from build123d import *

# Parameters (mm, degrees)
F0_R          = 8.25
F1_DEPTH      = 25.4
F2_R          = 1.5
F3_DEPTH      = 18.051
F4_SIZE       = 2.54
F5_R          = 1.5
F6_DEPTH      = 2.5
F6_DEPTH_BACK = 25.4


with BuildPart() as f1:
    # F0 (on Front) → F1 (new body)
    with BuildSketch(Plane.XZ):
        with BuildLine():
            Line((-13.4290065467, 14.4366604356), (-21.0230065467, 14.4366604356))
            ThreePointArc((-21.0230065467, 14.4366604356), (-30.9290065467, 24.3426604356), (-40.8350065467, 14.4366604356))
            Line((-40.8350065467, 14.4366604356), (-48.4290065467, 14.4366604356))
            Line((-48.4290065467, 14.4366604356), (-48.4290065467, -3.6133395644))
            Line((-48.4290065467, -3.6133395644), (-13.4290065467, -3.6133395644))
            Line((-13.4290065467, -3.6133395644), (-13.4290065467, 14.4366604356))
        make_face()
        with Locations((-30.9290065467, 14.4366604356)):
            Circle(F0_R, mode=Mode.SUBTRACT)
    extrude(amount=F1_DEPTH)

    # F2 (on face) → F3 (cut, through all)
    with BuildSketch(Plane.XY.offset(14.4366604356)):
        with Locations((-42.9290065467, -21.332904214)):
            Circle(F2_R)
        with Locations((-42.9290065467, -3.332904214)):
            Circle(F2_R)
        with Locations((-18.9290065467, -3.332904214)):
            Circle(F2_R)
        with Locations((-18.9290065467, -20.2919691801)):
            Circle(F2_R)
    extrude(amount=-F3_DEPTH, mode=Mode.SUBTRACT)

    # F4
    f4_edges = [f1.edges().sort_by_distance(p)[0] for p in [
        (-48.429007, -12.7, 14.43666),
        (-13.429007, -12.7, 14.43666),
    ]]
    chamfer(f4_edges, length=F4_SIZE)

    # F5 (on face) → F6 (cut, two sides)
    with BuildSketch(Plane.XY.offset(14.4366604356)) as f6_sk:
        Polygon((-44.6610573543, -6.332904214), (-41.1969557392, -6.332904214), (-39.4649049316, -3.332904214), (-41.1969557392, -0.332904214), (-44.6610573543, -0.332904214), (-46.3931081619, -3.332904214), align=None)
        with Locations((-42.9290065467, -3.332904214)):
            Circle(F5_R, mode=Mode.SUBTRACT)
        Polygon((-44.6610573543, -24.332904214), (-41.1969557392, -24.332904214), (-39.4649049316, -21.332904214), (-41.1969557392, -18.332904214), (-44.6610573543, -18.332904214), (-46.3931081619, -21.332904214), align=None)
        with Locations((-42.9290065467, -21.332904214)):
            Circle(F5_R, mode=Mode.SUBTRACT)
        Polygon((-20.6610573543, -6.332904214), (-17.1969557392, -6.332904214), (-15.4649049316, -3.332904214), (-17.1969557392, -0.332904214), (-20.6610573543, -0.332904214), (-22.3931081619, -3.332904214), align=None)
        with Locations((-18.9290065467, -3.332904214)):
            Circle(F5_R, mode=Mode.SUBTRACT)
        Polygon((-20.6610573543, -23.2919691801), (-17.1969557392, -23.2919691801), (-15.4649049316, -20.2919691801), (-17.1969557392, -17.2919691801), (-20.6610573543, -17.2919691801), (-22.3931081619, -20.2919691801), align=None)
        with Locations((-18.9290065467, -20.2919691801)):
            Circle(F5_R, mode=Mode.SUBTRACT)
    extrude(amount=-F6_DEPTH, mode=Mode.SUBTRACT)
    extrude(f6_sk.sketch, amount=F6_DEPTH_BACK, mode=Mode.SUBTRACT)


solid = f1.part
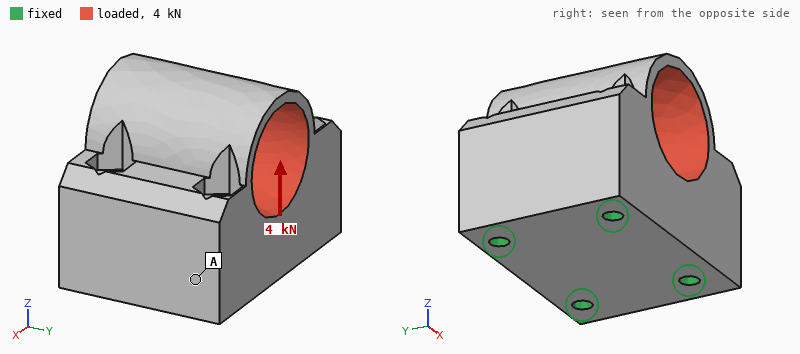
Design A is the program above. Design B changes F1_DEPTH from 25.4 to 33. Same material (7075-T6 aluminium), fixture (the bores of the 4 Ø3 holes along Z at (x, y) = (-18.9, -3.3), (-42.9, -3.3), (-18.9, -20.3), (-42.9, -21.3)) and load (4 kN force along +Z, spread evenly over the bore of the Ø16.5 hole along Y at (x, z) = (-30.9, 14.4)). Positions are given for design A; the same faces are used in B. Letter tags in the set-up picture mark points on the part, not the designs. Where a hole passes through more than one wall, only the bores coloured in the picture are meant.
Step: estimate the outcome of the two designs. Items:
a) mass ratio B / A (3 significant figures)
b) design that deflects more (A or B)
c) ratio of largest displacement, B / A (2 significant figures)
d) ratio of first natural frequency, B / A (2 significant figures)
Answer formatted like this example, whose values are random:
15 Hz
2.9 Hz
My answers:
1.32
A
0.73
1.0
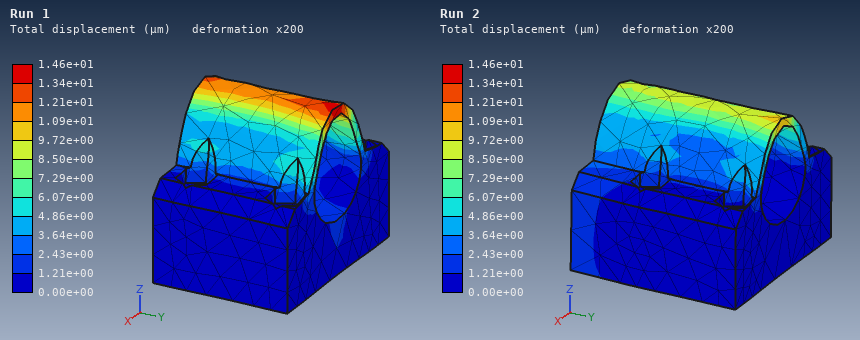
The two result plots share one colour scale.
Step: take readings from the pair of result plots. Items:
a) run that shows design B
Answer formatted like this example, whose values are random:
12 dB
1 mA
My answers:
Run 2
